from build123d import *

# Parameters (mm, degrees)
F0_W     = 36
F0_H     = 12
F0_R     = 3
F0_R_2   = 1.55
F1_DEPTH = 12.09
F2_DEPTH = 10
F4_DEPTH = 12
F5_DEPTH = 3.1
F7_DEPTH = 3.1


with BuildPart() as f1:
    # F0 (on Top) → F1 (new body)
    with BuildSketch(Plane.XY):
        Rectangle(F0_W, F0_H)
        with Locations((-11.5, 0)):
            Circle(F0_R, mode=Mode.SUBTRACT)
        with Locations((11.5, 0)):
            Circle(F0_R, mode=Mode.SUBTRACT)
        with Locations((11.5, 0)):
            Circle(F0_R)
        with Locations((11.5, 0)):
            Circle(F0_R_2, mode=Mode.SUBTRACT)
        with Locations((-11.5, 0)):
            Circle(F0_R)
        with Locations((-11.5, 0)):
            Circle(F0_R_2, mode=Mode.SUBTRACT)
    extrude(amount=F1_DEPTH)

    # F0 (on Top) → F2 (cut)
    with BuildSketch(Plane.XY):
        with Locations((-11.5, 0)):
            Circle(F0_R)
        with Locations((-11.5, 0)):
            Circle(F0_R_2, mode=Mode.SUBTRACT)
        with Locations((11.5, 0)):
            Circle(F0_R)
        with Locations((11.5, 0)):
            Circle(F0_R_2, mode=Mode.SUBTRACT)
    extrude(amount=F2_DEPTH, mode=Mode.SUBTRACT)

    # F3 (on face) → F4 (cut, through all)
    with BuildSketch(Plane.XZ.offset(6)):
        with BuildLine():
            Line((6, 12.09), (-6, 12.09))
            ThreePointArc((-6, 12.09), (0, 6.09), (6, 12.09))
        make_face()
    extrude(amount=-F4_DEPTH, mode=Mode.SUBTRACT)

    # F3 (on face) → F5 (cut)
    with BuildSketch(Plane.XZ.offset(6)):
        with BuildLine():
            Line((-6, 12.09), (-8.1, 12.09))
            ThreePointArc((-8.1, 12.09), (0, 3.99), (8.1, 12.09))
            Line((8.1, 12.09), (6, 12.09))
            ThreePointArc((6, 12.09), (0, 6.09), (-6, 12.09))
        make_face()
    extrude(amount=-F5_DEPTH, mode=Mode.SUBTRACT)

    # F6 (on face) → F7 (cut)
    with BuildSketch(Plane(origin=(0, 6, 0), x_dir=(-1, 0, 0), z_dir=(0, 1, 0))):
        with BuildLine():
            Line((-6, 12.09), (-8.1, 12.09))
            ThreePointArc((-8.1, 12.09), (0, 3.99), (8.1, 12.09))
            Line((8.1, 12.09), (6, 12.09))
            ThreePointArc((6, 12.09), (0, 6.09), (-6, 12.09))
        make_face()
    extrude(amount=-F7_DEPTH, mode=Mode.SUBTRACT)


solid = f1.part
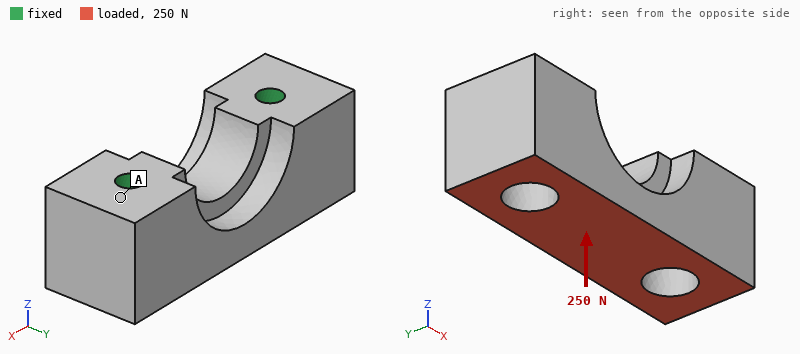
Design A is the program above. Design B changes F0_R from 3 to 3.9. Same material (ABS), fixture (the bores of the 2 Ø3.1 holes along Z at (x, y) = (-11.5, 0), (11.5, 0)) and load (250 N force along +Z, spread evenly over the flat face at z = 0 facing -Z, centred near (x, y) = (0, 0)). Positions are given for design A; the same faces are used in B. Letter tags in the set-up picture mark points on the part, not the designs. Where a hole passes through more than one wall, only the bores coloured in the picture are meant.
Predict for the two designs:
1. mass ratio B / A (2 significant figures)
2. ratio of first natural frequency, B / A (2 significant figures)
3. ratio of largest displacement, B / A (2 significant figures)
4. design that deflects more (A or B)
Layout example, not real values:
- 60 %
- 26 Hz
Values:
- 0.89
- 0.98
- 1.4
- B
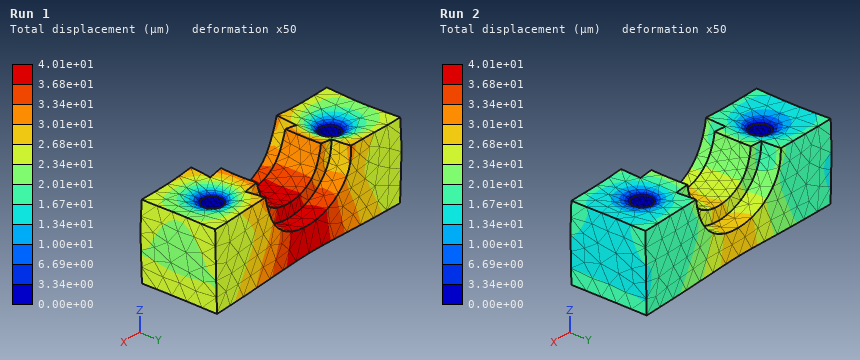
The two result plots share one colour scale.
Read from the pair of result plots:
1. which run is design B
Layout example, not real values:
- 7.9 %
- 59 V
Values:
- Run 1
